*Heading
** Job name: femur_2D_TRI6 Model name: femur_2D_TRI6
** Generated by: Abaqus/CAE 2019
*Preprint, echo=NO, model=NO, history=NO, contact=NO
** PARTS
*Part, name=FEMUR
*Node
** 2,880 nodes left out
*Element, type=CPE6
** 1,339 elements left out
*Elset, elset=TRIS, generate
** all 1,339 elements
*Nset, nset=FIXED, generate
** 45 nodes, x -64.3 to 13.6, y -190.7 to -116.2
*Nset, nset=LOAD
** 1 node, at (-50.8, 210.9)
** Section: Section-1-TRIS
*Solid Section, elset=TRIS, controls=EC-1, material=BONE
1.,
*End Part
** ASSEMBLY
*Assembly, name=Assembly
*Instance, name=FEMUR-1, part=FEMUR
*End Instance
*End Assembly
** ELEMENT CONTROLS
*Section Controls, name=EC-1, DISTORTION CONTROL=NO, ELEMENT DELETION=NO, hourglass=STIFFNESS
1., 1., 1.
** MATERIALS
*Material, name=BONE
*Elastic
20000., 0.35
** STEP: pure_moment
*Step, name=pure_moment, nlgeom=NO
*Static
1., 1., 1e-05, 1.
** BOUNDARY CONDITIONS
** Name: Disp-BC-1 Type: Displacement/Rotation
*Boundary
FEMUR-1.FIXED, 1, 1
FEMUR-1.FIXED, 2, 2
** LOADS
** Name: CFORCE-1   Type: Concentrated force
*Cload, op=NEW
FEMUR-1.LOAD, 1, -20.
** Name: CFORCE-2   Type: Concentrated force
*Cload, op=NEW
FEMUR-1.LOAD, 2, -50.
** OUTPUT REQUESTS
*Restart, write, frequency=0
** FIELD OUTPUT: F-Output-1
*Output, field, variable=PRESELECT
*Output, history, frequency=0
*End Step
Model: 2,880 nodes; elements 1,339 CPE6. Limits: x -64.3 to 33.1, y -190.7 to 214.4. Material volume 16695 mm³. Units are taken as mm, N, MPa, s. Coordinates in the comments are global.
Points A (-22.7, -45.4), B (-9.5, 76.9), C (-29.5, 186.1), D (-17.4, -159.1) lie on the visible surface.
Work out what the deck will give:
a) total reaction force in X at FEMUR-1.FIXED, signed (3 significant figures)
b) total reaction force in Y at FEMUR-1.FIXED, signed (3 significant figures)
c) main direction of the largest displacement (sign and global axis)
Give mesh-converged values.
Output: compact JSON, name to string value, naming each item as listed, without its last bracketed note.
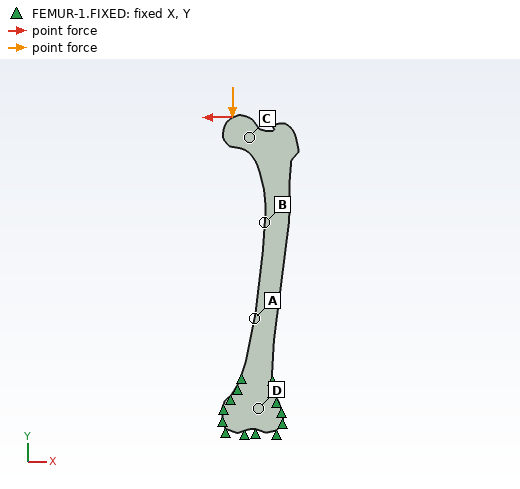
{"total reaction force in X at FEMUR-1.FIXED, signed": "20.0 N", "total reaction force in Y at FEMUR-1.FIXED, signed": "50.0 N", "main direction of the largest displacement": "-X"}
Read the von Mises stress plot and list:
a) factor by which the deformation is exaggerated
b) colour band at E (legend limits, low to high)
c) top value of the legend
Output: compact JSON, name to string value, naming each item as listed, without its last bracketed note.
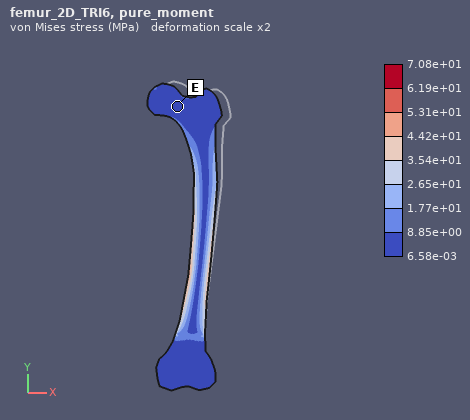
{"factor by which the deformation is exaggerated": "2", "colour band at E": "6.58e-03 to 8.85e+00 MPa", "top value of the legend": "7.08e+01 MPa"}
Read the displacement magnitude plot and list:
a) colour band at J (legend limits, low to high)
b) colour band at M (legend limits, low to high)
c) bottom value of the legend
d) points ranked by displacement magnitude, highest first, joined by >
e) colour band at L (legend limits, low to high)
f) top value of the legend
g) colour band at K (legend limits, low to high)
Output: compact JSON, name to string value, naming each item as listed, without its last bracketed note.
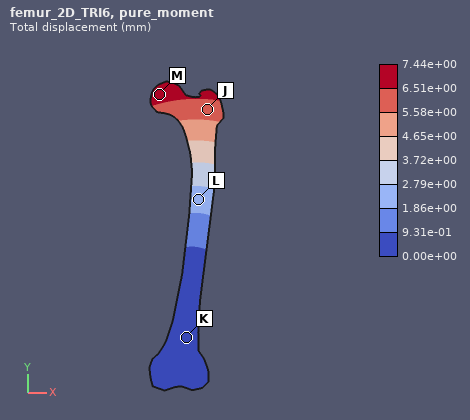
{"colour band at J": "5.58e+00 to 6.51e+00 mm", "colour band at M": "6.51e+00 to 7.44e+00 mm", "bottom value of the legend": "0.00e+00 mm", "points ranked by displacement magnitude, highest first, joined by >": "M > J > L > K", "colour band at L": "1.86e+00 to 2.79e+00 mm", "top value of the legend": "7.44e+00 mm", "colour band at K": "0.00e+00 to 9.31e-01 mm"}
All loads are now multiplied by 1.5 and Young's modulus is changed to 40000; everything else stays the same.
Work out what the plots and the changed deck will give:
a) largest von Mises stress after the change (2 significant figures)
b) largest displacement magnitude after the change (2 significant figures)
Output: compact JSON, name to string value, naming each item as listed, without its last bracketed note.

{"largest von Mises stress after the change": "110 MPa", "largest displacement magnitude after the change": "5.6 mm"}
